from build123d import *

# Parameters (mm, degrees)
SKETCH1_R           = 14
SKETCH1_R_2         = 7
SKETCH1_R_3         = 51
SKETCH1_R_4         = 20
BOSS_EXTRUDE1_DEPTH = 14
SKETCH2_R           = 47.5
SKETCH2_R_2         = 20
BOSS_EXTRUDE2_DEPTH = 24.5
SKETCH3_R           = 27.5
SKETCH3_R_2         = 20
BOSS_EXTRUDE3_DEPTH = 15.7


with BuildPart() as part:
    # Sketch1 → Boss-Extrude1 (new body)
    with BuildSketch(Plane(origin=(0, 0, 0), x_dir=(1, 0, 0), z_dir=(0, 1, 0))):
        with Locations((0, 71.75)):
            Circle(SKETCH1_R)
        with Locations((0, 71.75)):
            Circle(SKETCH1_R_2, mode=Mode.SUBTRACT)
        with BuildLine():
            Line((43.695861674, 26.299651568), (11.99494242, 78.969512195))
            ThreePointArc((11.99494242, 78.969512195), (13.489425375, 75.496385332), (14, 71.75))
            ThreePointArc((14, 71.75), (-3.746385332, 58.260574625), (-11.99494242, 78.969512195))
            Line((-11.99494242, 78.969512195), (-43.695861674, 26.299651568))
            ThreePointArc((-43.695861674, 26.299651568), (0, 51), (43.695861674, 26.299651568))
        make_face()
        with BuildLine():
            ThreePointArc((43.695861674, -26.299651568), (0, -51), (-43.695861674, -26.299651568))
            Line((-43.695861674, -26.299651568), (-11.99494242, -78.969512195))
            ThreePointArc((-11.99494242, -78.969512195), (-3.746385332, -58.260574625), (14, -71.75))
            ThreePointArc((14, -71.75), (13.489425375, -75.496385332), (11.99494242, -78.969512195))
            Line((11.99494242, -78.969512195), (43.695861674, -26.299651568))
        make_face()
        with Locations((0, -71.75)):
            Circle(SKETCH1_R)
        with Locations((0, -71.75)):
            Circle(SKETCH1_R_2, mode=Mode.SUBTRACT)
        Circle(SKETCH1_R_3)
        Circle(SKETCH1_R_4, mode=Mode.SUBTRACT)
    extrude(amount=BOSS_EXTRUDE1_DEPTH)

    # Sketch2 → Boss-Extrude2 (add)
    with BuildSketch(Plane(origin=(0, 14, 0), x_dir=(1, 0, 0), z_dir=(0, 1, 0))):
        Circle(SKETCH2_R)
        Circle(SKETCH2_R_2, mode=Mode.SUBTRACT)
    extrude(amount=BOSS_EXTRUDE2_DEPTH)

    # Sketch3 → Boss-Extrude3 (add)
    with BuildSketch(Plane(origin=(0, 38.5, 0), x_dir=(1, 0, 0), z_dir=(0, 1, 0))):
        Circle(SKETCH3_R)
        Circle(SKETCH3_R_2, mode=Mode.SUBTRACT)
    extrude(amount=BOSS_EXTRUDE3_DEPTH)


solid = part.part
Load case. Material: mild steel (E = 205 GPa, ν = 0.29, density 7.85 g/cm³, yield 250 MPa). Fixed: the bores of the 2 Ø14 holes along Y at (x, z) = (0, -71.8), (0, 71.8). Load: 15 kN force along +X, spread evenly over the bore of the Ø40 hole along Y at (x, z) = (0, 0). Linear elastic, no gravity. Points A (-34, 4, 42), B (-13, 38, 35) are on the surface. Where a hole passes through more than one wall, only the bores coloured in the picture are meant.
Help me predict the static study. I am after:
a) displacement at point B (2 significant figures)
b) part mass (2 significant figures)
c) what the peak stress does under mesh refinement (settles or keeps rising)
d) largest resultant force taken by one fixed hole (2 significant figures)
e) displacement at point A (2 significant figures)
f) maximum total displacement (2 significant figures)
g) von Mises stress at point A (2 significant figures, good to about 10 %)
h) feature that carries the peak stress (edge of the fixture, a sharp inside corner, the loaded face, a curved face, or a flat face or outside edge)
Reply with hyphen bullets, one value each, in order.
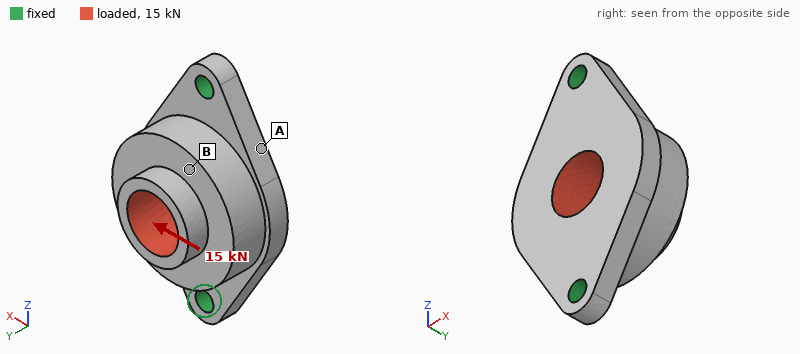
- 47 µm
- 2.3 kg
- keeps rising
- 7.5 kN
- 38 µm
- 74 µm
- 30 MPa
- edge of the fixture
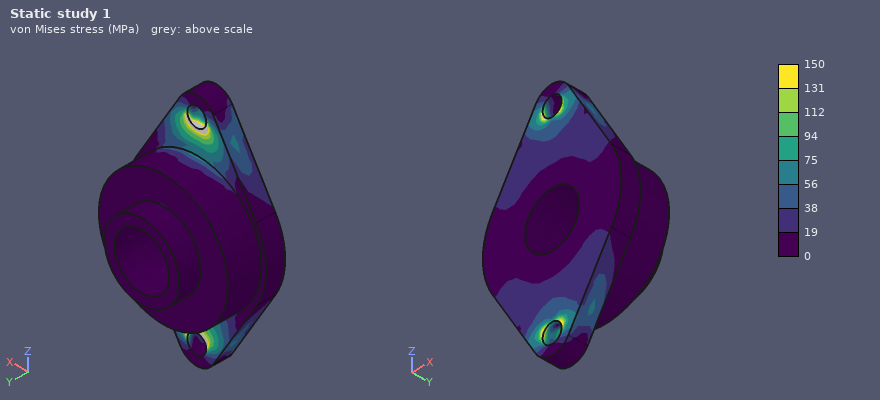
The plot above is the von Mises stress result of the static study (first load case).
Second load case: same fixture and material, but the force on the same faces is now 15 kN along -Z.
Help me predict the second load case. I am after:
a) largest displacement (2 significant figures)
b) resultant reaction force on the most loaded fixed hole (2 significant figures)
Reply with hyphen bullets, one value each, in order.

- 7.7 µm
- 7.9 kN
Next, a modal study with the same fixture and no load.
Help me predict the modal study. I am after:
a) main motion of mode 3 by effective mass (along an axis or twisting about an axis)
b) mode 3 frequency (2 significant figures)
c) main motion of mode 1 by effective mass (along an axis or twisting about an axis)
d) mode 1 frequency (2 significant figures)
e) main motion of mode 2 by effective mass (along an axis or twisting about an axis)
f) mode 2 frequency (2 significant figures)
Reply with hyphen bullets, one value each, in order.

- along X
- 5900 Hz
- along X
- 1700 Hz
- along Y
- 3300 Hz
